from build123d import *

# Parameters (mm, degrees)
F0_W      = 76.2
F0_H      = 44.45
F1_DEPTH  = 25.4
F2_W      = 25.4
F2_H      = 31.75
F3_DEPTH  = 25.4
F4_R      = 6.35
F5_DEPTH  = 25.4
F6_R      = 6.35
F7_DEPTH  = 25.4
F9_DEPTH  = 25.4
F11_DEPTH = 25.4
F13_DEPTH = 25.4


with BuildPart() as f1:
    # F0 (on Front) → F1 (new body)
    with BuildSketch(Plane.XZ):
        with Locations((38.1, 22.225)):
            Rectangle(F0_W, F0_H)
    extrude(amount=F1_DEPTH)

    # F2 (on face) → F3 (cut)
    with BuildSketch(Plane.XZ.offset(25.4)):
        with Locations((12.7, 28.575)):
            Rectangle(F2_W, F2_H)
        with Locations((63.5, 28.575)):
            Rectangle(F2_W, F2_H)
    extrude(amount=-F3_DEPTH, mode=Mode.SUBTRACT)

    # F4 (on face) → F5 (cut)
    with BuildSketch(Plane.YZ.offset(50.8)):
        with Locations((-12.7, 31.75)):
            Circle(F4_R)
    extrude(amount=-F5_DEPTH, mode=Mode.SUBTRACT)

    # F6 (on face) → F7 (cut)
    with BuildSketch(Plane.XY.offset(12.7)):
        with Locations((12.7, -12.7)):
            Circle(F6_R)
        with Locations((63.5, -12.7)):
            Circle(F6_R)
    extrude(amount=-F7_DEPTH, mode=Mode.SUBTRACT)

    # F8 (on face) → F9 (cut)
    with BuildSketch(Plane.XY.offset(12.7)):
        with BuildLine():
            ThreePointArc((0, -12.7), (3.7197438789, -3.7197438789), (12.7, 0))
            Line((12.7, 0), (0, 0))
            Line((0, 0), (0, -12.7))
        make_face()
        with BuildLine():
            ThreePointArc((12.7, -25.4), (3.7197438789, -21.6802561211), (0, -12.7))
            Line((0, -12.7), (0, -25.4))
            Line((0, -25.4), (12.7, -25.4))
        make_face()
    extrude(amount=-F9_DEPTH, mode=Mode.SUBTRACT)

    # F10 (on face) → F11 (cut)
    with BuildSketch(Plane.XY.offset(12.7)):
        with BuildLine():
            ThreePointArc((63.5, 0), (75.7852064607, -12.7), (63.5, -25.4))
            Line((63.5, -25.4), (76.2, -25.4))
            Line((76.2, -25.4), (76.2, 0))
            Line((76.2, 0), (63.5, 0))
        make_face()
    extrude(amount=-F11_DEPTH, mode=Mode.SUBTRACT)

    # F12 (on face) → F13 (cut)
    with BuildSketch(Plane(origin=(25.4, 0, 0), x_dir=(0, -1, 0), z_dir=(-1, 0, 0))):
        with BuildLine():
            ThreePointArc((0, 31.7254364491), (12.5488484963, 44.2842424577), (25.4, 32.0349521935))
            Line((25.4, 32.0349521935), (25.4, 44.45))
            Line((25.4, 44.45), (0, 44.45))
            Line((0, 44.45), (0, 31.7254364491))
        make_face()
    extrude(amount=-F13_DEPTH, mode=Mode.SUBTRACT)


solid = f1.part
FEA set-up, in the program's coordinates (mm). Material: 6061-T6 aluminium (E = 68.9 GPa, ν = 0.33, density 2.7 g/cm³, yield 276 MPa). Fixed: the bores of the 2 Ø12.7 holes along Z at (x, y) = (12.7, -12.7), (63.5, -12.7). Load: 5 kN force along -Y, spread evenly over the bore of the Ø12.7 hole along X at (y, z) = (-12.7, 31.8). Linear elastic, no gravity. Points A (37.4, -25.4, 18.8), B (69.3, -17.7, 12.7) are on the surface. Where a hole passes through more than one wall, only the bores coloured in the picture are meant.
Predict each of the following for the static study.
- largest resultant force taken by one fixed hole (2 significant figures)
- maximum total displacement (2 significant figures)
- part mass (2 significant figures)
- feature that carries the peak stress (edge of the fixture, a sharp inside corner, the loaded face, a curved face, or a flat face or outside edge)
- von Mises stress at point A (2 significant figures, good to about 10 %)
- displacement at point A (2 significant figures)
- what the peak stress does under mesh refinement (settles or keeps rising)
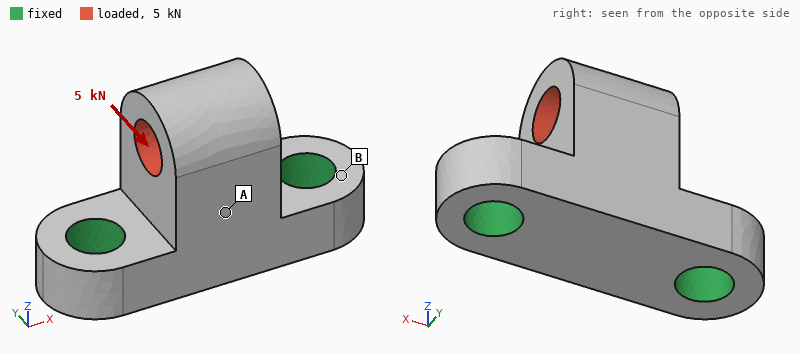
2.5 kN
0.11 mm
94 g
edge of the fixture
23 MPa
0.047 mm
keeps rising
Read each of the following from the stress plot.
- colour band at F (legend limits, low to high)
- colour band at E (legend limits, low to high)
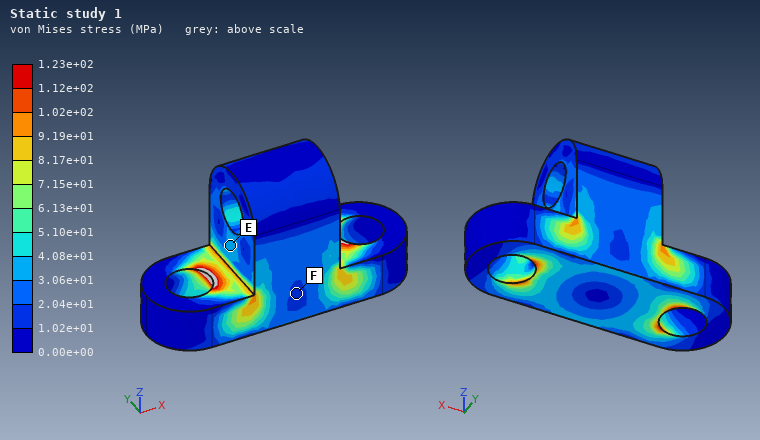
1.02e+01 to 2.04e+01 MPa
3.06e+01 to 4.08e+01 MPa
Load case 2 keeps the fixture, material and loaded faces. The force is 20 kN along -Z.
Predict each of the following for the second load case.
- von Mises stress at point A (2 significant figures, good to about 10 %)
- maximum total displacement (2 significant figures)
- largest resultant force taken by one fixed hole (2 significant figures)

26 MPa
46 µm
10 kN
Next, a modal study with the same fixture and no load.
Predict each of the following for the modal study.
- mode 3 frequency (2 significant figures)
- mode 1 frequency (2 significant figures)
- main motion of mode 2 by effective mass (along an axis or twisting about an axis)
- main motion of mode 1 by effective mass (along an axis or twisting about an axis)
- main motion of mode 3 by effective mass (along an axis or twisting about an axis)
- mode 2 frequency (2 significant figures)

17 kHz
7000 Hz
along X
along Y
along Z
12 kHz
